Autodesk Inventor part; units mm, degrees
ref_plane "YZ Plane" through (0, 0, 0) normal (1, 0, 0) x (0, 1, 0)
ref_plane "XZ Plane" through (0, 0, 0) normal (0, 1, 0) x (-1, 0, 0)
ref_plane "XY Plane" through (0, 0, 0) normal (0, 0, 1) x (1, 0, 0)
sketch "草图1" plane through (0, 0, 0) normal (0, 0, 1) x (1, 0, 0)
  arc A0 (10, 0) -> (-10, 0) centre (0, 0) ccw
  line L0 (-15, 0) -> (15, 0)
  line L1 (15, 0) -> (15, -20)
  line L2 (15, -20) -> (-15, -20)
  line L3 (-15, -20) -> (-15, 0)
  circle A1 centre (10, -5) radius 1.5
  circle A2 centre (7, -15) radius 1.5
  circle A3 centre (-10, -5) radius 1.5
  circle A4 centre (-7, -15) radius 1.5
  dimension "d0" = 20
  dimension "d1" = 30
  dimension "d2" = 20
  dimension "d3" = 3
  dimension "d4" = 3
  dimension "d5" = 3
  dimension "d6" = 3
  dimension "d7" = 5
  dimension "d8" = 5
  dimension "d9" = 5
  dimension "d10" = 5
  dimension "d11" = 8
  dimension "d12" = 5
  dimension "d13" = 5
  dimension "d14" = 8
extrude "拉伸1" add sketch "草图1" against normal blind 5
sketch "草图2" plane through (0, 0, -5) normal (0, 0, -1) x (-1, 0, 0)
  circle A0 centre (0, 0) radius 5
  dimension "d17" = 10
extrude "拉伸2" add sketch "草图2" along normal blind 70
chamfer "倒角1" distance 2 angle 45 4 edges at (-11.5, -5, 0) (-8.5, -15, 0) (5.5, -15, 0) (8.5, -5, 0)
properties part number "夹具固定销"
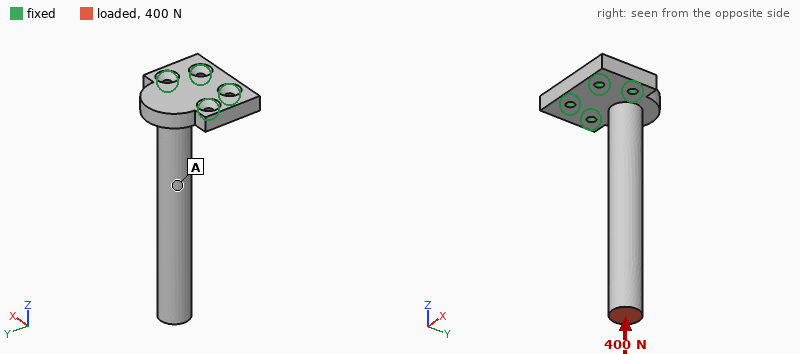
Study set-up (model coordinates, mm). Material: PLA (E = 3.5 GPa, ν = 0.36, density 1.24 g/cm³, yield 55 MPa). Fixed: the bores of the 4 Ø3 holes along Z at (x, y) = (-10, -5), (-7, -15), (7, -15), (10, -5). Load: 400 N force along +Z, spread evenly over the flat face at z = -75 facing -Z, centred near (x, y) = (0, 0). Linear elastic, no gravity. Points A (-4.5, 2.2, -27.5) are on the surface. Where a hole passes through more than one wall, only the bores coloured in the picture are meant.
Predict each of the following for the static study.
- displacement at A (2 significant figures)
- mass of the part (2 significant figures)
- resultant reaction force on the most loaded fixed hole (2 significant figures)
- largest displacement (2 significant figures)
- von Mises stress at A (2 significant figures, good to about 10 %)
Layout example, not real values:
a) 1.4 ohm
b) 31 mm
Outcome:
a) 0.38 mm
b) 11 g
c) 240 N
d) 1.0 mm
e) 5.1 MPa
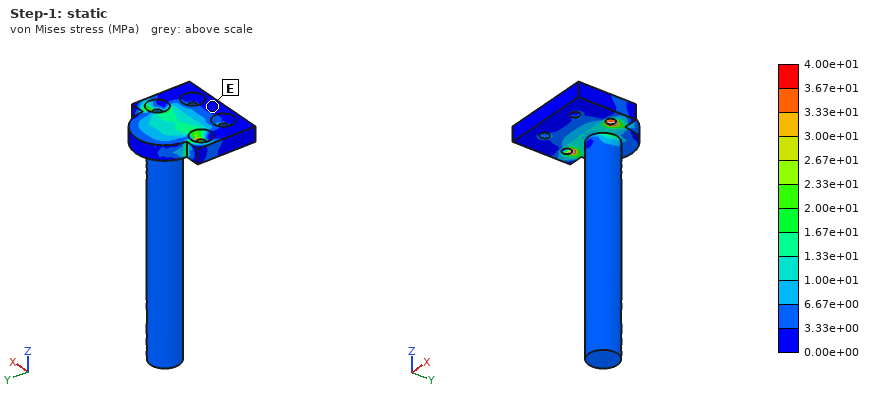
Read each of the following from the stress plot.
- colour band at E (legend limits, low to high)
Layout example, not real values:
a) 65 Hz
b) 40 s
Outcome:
a) 0.00e+00 to 3.33e+00 MPa
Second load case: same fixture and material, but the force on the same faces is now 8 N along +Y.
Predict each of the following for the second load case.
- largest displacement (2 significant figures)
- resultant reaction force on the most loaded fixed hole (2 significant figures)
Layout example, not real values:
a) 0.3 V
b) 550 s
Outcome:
a) 0.88 mm
b) 22 N
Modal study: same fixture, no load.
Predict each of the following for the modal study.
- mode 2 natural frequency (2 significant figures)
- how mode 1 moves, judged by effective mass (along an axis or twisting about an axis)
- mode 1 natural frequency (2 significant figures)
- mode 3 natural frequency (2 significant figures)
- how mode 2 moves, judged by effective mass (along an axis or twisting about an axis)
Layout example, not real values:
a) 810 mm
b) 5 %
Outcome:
a) 410 Hz
b) along Y
c) 350 Hz
d) 2200 Hz
e) along X
